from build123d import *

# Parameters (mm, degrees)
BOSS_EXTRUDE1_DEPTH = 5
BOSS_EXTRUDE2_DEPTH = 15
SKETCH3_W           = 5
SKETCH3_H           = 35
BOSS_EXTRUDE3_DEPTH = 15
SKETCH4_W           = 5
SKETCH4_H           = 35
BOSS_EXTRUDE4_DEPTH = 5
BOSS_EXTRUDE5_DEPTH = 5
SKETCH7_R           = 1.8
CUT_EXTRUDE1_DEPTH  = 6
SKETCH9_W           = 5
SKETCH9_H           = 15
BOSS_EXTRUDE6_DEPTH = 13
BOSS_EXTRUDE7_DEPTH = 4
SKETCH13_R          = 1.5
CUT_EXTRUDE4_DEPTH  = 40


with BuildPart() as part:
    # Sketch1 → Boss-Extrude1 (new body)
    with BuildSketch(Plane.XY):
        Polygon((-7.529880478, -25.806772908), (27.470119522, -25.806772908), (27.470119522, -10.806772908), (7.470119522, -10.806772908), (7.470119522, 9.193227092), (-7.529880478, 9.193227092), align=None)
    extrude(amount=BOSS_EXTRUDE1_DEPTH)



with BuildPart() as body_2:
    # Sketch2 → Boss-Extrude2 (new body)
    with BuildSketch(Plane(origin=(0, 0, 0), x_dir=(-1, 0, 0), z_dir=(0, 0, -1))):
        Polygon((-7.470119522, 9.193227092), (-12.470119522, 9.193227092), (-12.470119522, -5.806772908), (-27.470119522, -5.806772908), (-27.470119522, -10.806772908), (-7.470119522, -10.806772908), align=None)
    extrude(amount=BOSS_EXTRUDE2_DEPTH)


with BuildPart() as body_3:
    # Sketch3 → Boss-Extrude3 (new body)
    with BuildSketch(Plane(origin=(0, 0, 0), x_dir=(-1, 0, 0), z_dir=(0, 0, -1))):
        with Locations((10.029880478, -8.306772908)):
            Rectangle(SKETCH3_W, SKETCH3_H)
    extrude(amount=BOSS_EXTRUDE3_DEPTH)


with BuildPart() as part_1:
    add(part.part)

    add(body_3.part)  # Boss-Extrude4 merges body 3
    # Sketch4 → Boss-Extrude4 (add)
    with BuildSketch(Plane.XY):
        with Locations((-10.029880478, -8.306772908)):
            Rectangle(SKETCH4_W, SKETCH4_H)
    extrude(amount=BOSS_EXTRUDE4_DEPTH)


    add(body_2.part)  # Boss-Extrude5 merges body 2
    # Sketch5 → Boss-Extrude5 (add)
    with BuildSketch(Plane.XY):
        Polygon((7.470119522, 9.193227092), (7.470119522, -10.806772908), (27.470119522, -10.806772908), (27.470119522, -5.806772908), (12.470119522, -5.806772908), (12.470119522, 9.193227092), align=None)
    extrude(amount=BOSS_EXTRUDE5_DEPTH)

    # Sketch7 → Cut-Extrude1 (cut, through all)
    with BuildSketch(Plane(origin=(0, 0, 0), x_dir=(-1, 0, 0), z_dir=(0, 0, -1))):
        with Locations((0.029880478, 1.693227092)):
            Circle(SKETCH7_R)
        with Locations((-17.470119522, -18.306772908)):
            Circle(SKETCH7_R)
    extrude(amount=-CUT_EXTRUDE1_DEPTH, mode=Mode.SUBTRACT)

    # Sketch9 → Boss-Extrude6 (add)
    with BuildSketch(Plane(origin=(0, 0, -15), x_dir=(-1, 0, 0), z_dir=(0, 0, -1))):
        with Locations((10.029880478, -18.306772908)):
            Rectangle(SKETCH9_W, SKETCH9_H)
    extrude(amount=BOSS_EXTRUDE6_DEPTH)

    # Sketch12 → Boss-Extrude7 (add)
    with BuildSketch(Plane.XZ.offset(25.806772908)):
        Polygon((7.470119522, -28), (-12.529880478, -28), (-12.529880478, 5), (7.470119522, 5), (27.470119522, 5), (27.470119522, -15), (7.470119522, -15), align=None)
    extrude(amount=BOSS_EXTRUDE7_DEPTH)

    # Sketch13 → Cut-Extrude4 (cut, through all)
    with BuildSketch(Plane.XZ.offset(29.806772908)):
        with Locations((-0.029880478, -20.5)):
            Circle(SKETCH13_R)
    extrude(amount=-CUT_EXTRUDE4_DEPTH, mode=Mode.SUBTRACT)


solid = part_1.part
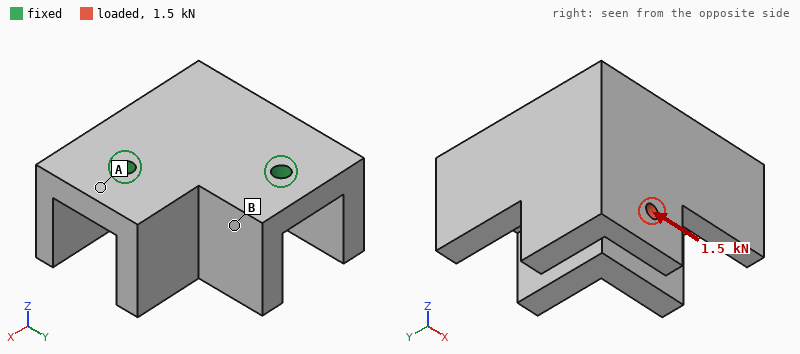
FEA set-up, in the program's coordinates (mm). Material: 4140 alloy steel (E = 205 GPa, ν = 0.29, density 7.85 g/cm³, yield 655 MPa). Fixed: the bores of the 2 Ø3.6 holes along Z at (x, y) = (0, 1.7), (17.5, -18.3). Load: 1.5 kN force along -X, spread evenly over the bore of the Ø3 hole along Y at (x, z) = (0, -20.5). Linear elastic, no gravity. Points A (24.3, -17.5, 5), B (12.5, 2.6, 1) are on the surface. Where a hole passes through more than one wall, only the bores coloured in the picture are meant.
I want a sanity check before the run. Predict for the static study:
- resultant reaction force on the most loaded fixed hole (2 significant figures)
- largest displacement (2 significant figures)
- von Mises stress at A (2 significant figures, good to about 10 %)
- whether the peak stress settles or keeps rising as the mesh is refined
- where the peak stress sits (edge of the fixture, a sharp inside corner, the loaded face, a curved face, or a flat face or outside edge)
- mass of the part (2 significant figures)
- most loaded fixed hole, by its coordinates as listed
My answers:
1.8 kN
0.13 mm
89 MPa
keeps rising
edge of the fixture
130 g
(17.5, -18.3)
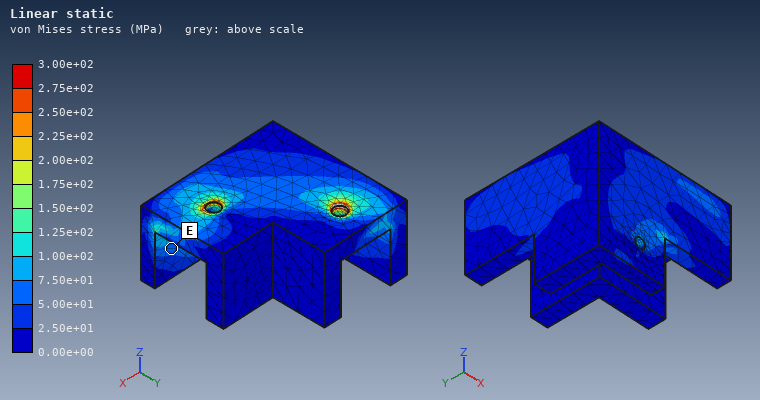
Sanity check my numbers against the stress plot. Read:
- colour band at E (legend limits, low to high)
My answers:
5.00e+01 to 7.50e+01 MPa
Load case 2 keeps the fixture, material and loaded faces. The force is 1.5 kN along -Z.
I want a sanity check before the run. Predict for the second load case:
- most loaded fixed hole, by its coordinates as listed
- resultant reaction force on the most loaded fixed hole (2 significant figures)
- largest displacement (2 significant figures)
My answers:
(17.5, -18.3)
1.1 kN
0.10 mm
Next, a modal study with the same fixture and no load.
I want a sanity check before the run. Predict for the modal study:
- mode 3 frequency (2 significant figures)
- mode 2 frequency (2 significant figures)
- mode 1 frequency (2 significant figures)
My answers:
9000 Hz
6400 Hz
2900 Hz
